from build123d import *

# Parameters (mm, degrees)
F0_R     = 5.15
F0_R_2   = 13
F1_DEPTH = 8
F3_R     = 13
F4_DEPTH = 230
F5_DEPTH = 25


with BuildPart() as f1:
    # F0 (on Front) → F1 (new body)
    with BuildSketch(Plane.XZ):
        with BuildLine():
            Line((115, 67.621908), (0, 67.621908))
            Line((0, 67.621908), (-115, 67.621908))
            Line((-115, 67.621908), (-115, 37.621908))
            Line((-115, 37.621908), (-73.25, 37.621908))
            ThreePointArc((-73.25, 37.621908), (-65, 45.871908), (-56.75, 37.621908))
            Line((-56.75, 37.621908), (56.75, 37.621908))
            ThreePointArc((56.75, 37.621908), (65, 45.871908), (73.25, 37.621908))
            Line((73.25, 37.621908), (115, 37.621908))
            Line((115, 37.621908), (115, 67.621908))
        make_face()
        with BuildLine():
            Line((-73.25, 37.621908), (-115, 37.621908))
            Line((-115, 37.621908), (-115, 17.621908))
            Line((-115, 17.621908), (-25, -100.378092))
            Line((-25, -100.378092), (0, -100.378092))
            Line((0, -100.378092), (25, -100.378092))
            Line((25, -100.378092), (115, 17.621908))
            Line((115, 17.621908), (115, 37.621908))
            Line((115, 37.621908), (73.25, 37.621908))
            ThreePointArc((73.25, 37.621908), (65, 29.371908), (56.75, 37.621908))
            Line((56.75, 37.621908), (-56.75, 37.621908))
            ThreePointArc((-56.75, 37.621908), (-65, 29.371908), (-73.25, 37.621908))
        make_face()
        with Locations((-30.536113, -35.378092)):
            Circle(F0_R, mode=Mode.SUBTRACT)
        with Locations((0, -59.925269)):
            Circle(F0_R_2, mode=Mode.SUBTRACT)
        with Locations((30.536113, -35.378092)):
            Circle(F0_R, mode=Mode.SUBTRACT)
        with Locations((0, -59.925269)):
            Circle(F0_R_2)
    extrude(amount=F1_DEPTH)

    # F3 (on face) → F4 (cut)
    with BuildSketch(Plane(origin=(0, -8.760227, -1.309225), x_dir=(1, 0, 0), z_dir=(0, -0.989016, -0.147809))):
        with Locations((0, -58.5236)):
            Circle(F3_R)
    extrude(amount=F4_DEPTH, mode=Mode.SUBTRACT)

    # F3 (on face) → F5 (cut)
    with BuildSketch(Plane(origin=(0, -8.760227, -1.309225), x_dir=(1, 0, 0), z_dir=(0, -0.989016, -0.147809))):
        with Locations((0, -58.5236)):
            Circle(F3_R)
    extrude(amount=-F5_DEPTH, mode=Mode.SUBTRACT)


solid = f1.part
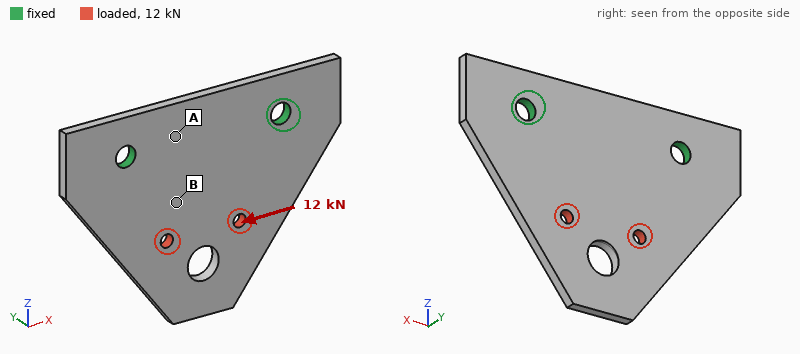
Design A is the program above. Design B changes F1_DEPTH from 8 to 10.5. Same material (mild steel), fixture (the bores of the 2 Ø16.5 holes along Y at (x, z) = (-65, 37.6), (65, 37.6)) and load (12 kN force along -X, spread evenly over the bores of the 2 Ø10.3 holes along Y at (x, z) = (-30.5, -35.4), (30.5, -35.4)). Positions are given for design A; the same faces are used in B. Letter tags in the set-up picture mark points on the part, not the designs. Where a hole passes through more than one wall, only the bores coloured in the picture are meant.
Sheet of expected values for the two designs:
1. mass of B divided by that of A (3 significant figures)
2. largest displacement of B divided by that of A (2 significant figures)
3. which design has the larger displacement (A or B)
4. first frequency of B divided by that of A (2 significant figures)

1.31
0.76
A
1.3
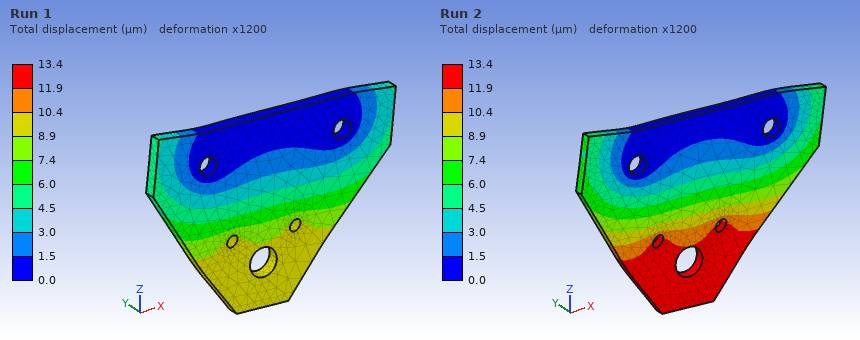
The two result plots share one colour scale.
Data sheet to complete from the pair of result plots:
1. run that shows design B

Run 1
